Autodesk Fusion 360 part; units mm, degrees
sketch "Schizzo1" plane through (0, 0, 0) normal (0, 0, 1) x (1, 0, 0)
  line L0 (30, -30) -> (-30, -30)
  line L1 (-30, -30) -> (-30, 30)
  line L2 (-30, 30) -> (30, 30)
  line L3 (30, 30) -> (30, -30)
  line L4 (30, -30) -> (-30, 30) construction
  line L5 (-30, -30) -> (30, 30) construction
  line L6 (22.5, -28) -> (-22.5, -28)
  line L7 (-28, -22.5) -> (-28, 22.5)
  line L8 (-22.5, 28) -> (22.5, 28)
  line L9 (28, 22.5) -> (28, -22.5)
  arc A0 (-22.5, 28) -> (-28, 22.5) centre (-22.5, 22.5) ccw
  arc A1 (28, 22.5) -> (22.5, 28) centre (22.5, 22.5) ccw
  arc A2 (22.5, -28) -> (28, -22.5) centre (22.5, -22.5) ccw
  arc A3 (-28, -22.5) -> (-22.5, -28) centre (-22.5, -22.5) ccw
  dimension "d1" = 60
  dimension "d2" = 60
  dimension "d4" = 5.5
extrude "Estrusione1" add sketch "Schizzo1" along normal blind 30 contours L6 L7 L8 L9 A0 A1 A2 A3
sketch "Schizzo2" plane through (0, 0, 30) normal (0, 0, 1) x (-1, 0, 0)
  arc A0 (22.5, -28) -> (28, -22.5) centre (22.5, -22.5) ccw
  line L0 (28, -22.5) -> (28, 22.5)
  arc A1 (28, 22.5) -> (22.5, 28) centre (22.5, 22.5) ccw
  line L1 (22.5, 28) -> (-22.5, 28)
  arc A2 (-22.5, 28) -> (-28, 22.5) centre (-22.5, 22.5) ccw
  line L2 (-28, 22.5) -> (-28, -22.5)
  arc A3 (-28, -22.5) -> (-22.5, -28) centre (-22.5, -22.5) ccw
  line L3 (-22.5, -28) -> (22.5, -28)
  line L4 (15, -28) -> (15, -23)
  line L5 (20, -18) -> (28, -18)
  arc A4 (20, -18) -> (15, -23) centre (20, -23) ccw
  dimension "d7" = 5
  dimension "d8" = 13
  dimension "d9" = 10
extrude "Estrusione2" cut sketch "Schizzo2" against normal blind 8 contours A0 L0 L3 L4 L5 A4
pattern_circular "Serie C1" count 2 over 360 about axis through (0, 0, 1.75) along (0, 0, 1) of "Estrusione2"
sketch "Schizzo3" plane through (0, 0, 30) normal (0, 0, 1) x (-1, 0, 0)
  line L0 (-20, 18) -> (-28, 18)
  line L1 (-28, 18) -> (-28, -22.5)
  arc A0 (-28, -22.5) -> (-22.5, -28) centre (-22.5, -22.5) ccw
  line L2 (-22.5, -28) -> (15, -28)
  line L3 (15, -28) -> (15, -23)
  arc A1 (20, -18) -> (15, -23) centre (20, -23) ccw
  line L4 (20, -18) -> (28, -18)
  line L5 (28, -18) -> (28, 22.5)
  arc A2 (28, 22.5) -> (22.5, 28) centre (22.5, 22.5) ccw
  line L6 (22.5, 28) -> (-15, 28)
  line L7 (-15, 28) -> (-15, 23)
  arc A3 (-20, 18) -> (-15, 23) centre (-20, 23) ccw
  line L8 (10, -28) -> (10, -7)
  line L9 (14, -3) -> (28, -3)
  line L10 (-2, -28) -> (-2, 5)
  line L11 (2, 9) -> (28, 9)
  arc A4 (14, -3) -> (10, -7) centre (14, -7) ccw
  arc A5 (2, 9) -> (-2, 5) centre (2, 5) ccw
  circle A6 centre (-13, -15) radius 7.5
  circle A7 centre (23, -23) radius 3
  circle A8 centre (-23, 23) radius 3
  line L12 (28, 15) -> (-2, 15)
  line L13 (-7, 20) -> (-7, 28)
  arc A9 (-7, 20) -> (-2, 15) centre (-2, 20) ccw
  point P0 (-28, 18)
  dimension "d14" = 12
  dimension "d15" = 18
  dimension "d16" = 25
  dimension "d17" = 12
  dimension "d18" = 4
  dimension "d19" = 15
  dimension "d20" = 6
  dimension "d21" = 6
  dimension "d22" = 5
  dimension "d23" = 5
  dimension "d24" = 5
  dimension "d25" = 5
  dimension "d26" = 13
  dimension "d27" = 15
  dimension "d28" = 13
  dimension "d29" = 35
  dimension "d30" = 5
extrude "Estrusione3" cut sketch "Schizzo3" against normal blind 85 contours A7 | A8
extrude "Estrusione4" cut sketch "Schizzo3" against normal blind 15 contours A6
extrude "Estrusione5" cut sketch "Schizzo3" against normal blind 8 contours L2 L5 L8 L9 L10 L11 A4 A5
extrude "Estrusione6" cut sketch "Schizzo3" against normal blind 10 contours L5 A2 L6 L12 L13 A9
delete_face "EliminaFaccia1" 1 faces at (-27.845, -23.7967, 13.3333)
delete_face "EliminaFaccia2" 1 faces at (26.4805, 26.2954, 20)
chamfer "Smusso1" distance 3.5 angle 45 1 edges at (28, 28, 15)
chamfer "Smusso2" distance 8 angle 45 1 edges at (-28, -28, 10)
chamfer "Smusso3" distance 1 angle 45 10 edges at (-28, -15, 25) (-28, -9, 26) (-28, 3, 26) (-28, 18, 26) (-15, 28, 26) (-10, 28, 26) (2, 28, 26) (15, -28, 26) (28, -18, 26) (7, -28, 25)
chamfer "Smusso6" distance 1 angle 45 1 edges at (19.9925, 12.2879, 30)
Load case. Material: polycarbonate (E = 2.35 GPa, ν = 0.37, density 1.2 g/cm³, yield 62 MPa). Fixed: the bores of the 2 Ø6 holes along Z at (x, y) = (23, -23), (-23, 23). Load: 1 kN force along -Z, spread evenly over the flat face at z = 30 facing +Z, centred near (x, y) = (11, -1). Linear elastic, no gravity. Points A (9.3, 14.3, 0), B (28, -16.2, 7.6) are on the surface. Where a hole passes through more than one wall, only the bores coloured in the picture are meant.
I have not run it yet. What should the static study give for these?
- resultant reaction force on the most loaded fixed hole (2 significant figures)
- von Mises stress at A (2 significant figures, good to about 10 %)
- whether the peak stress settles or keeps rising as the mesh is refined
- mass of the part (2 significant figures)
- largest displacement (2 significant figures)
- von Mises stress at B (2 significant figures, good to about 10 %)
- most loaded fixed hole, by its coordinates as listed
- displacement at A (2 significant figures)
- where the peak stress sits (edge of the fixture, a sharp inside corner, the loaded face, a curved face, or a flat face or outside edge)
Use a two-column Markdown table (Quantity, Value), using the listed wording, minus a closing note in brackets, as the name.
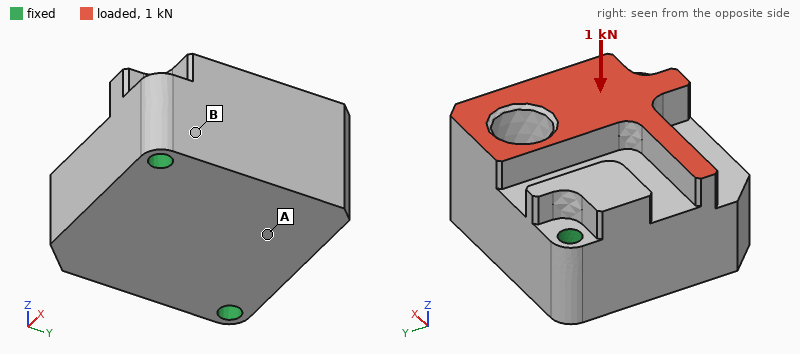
| Quantity | Value |
|---|---|
| resultant reaction force on the most loaded fixed hole | 640 N |
| von Mises stress at A | 1.4 MPa |
| whether the peak stress settles or keeps rising as the mesh is refined | keeps rising |
| mass of the part | 93 g |
| largest displacement | 0.13 mm |
| von Mises stress at B | 3.8 MPa |
| most loaded fixed hole, by its coordinates as listed | (23, -23) |
| displacement at A | 0.065 mm |
| where the peak stress sits | edge of the fixture |
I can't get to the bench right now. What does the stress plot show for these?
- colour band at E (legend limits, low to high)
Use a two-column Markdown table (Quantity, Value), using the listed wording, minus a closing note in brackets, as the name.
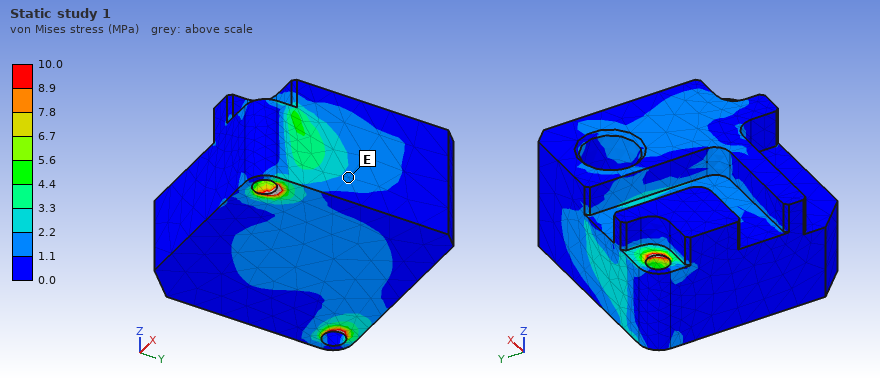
| Quantity | Value |
|---|---|
| colour band at E | 1.1 to 2.2 MPa |
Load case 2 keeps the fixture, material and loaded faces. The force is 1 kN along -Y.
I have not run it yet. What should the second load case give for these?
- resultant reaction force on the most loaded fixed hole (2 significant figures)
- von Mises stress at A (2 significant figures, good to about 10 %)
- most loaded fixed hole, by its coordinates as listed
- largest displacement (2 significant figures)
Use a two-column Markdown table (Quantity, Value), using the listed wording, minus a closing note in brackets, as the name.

| Quantity | Value |
|---|---|
| resultant reaction force on the most loaded fixed hole | 730 N |
| von Mises stress at A | 1.2 MPa |
| most loaded fixed hole, by its coordinates as listed | (23, -23) |
| largest displacement | 0.17 mm |
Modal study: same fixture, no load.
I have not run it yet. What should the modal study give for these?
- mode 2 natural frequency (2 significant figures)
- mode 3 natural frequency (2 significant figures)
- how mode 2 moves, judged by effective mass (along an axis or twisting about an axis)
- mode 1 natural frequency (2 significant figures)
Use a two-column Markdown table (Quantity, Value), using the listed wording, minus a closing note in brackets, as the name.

| Quantity | Value |
|---|---|
| mode 2 natural frequency | 2800 Hz |
| mode 3 natural frequency | 3900 Hz |
| how mode 2 moves, judged by effective mass | along Z |
| mode 1 natural frequency | 2000 Hz |
